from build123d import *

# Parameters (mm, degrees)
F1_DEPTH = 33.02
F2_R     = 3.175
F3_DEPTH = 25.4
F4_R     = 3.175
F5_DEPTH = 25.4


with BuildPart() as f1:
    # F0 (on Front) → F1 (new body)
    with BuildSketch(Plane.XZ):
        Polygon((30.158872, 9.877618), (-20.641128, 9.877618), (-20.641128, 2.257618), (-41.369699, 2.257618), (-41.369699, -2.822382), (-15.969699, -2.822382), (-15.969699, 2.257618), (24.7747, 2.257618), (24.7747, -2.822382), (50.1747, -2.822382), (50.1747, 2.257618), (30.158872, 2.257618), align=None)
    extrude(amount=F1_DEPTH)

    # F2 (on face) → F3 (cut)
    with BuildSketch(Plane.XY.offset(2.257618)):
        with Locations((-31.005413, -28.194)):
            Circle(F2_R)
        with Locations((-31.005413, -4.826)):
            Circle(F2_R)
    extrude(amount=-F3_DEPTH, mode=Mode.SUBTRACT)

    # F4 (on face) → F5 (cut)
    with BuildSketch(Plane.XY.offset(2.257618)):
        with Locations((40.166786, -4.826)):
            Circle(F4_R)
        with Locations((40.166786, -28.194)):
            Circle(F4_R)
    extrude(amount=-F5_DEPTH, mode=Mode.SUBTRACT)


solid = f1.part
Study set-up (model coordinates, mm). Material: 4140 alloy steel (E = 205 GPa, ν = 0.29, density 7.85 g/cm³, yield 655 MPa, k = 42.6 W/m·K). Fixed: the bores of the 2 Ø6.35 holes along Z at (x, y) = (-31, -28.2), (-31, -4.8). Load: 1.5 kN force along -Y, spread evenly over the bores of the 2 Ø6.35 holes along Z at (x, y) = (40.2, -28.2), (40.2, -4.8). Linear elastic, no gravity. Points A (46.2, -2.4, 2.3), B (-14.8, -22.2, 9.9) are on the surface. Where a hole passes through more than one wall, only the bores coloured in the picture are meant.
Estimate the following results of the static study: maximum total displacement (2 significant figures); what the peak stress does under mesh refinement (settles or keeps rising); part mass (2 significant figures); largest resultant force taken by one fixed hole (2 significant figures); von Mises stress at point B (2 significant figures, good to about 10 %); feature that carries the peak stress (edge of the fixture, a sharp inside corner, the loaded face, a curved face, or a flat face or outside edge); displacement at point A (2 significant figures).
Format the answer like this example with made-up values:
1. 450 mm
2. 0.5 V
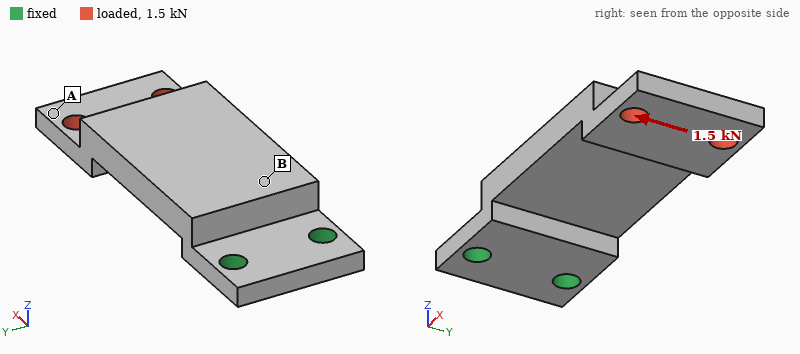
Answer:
1. 0.15 mm
2. keeps rising
3. 160 g
4. 4.3 kN
5. 88 MPa
6. a sharp inside corner
7. 0.13 mm
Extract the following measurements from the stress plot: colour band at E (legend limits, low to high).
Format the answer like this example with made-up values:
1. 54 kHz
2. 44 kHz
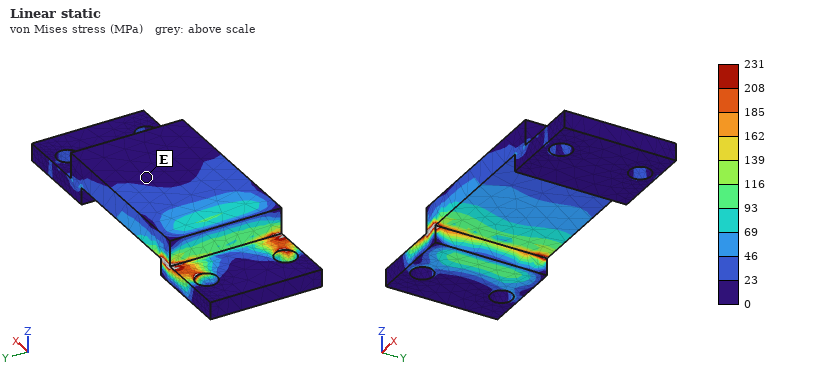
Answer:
1. 0 to 23 MPa
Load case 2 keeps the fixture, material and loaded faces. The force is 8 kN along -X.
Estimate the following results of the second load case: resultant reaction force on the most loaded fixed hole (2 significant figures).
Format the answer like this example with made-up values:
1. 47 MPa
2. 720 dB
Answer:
1. 4.0 kN
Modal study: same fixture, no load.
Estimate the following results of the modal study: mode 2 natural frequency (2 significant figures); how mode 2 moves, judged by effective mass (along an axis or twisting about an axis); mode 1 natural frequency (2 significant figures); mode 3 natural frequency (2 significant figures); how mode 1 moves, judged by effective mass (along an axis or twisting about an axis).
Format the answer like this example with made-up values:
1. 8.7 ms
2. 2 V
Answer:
1. 2600 Hz
2. along Y
3. 700 Hz
4. 4600 Hz
5. along Z
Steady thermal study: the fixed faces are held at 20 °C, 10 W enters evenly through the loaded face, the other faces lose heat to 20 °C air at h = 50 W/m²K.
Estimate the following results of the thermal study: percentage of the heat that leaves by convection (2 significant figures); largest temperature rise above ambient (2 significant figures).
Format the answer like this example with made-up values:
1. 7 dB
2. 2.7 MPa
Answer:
1. 69 %
2. 46 K
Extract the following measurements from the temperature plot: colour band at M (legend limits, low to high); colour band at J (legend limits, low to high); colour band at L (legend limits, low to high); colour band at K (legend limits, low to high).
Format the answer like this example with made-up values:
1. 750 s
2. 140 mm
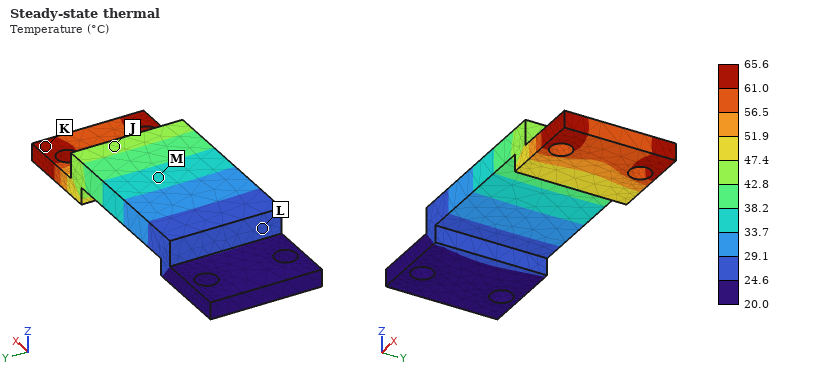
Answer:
1. 33.7 to 38.2 °C
2. 42.8 to 47.4 °C
3. 24.6 to 29.1 °C
4. 61.0 to 65.6 °C
